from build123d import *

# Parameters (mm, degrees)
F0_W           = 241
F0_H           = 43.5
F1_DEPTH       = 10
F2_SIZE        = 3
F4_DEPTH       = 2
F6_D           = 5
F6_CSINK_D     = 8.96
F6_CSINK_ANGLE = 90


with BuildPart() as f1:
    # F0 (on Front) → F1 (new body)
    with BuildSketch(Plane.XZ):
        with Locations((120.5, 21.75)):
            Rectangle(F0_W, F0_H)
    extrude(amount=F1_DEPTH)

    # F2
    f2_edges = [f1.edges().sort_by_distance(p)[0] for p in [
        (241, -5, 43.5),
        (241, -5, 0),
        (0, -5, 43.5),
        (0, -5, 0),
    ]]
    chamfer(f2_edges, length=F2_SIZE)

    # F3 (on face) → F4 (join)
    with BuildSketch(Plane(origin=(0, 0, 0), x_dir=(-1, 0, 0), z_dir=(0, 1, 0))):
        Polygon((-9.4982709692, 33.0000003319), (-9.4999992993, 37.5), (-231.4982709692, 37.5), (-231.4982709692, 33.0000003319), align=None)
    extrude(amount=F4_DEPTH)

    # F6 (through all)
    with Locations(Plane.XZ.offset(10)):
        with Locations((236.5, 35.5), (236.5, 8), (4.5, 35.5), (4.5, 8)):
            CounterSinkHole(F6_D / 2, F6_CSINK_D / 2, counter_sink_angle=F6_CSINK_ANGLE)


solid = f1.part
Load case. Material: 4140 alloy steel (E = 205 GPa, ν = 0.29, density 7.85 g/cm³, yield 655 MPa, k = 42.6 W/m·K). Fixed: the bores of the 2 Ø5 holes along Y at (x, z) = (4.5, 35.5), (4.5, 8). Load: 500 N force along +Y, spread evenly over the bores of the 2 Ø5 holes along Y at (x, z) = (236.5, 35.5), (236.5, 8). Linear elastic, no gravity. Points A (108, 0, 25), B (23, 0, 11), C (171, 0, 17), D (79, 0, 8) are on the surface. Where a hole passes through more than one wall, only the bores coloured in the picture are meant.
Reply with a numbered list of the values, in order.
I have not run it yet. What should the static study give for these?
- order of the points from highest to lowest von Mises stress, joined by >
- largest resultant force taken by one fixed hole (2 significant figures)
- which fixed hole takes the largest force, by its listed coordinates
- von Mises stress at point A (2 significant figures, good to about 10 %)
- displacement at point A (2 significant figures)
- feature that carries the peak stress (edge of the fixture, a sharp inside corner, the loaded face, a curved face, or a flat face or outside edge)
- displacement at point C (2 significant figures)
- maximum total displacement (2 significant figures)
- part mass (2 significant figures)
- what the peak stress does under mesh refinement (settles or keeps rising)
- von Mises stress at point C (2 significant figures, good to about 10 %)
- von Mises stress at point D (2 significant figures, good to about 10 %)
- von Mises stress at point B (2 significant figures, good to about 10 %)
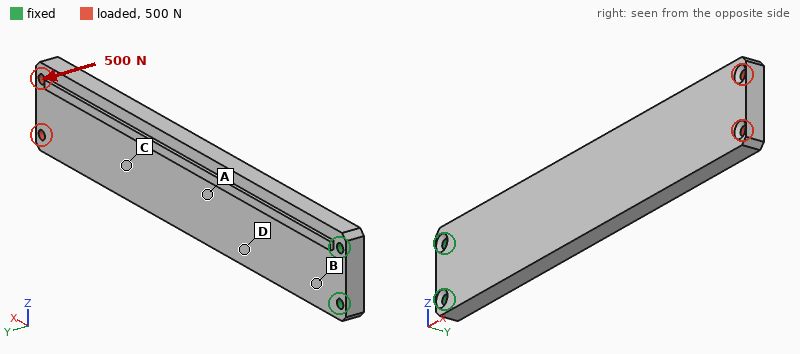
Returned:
1. B > D > A > C
2. 280 N
3. (4.5, 8)
4. 79 MPa
5. 0.73 mm
6. edge of the fixture
7. 1.6 mm
8. 2.8 mm
9. 830 g
10. keeps rising
11. 41 MPa
12. 100 MPa
13. 130 MPa
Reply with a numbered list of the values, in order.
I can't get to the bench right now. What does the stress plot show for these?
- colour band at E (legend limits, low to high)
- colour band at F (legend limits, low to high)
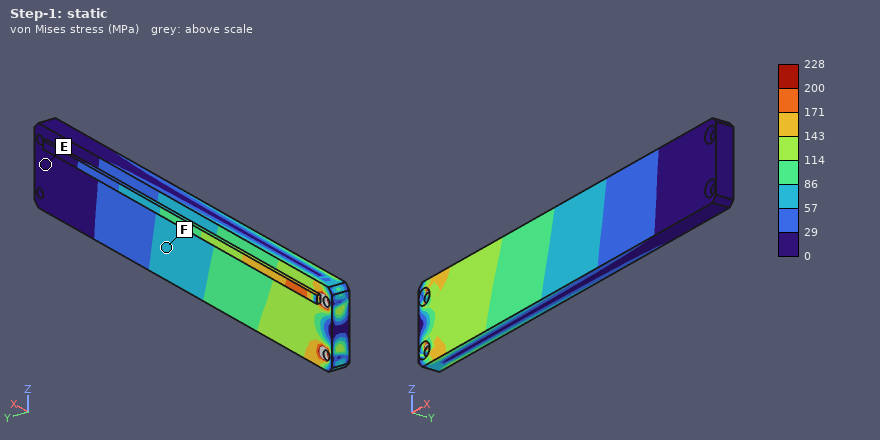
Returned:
1. 0 to 29 MPa
2. 57 to 86 MPa
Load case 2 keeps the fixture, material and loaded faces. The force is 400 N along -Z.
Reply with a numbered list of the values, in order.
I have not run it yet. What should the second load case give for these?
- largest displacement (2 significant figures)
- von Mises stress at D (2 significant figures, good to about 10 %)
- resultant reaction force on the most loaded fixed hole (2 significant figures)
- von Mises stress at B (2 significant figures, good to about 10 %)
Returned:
1. 0.13 mm
2. 13 MPa
3. 3.1 kN
4. 16 MPa
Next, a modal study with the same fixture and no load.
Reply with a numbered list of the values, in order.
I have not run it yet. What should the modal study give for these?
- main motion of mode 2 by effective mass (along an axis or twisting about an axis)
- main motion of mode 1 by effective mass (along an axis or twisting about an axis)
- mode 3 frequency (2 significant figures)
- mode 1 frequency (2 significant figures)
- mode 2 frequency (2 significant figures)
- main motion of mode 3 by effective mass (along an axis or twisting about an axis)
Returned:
1. along Z
2. along Y
3. 920 Hz
4. 150 Hz
5. 620 Hz
6. along Y
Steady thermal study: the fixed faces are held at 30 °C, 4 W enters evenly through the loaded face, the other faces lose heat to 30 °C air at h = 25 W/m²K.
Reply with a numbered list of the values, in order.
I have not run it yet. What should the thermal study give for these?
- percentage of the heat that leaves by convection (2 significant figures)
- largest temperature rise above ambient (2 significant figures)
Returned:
1. 89 %
2. 18 K
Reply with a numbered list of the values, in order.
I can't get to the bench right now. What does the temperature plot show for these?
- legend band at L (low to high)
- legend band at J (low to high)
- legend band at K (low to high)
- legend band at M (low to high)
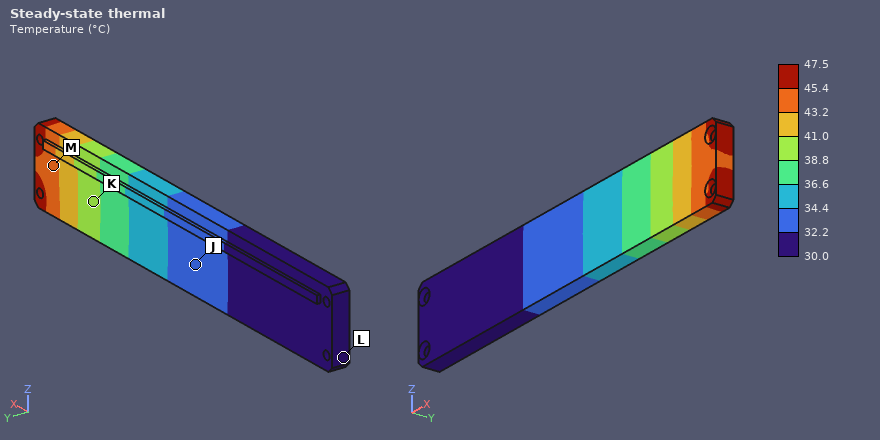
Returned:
1. 30.0 to 32.2 °C
2. 32.2 to 34.4 °C
3. 38.8 to 41.0 °C
4. 43.2 to 45.4 °C
